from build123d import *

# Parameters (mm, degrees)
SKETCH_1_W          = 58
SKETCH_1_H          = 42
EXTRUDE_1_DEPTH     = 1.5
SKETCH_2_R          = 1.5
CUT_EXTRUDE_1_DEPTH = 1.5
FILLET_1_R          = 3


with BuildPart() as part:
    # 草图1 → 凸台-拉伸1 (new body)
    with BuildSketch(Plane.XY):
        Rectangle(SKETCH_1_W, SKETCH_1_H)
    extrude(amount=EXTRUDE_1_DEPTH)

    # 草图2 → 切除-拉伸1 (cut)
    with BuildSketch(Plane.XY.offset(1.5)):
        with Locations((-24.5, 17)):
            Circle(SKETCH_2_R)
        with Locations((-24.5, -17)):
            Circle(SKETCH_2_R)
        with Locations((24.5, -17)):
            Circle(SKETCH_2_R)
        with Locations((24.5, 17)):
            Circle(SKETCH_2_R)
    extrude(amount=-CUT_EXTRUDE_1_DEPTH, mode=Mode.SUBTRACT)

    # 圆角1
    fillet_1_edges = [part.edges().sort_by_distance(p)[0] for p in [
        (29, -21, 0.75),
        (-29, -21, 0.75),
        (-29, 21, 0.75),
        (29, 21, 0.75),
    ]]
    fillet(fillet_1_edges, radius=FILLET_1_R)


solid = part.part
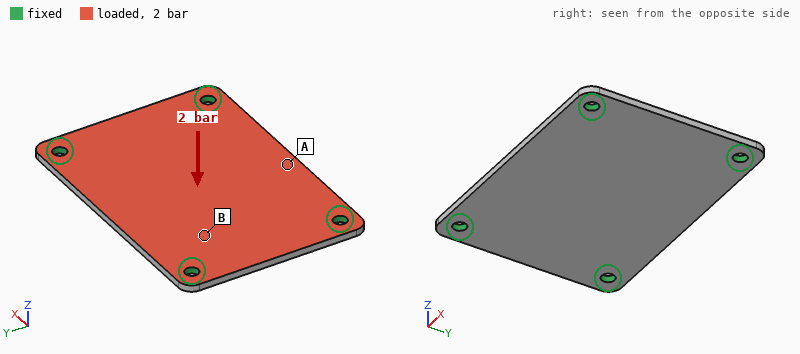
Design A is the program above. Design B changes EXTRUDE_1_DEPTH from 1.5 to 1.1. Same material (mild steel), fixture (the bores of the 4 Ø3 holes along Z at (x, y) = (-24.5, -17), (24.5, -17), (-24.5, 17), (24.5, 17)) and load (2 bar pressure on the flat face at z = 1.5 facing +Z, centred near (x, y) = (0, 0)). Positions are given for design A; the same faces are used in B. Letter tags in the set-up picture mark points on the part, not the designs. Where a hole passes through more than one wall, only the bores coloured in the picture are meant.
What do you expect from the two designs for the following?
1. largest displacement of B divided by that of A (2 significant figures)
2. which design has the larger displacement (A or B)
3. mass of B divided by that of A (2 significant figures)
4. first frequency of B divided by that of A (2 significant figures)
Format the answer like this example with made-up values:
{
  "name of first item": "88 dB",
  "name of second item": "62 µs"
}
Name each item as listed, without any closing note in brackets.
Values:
{
  "largest displacement of B divided by that of A": "2.5",
  "which design has the larger displacement": "B",
  "mass of B divided by that of A": "0.73",
  "first frequency of B divided by that of A": "0.74"
}
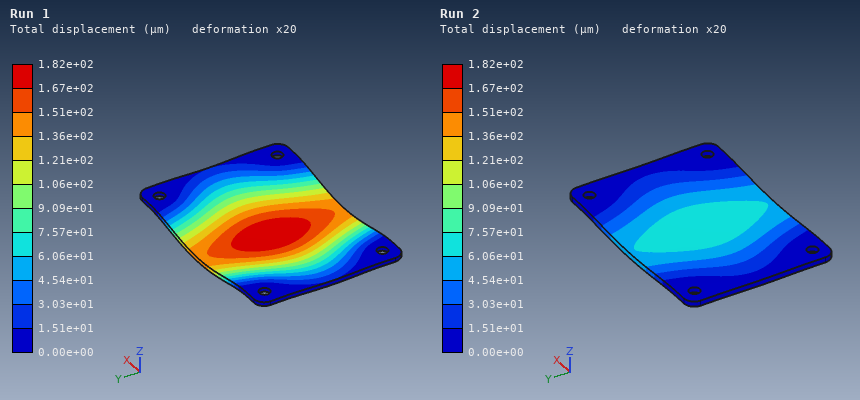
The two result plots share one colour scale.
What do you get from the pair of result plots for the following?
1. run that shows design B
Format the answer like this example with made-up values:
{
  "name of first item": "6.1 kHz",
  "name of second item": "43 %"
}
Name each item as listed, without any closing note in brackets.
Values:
{
  "run that shows design B": "Run 1"
}
